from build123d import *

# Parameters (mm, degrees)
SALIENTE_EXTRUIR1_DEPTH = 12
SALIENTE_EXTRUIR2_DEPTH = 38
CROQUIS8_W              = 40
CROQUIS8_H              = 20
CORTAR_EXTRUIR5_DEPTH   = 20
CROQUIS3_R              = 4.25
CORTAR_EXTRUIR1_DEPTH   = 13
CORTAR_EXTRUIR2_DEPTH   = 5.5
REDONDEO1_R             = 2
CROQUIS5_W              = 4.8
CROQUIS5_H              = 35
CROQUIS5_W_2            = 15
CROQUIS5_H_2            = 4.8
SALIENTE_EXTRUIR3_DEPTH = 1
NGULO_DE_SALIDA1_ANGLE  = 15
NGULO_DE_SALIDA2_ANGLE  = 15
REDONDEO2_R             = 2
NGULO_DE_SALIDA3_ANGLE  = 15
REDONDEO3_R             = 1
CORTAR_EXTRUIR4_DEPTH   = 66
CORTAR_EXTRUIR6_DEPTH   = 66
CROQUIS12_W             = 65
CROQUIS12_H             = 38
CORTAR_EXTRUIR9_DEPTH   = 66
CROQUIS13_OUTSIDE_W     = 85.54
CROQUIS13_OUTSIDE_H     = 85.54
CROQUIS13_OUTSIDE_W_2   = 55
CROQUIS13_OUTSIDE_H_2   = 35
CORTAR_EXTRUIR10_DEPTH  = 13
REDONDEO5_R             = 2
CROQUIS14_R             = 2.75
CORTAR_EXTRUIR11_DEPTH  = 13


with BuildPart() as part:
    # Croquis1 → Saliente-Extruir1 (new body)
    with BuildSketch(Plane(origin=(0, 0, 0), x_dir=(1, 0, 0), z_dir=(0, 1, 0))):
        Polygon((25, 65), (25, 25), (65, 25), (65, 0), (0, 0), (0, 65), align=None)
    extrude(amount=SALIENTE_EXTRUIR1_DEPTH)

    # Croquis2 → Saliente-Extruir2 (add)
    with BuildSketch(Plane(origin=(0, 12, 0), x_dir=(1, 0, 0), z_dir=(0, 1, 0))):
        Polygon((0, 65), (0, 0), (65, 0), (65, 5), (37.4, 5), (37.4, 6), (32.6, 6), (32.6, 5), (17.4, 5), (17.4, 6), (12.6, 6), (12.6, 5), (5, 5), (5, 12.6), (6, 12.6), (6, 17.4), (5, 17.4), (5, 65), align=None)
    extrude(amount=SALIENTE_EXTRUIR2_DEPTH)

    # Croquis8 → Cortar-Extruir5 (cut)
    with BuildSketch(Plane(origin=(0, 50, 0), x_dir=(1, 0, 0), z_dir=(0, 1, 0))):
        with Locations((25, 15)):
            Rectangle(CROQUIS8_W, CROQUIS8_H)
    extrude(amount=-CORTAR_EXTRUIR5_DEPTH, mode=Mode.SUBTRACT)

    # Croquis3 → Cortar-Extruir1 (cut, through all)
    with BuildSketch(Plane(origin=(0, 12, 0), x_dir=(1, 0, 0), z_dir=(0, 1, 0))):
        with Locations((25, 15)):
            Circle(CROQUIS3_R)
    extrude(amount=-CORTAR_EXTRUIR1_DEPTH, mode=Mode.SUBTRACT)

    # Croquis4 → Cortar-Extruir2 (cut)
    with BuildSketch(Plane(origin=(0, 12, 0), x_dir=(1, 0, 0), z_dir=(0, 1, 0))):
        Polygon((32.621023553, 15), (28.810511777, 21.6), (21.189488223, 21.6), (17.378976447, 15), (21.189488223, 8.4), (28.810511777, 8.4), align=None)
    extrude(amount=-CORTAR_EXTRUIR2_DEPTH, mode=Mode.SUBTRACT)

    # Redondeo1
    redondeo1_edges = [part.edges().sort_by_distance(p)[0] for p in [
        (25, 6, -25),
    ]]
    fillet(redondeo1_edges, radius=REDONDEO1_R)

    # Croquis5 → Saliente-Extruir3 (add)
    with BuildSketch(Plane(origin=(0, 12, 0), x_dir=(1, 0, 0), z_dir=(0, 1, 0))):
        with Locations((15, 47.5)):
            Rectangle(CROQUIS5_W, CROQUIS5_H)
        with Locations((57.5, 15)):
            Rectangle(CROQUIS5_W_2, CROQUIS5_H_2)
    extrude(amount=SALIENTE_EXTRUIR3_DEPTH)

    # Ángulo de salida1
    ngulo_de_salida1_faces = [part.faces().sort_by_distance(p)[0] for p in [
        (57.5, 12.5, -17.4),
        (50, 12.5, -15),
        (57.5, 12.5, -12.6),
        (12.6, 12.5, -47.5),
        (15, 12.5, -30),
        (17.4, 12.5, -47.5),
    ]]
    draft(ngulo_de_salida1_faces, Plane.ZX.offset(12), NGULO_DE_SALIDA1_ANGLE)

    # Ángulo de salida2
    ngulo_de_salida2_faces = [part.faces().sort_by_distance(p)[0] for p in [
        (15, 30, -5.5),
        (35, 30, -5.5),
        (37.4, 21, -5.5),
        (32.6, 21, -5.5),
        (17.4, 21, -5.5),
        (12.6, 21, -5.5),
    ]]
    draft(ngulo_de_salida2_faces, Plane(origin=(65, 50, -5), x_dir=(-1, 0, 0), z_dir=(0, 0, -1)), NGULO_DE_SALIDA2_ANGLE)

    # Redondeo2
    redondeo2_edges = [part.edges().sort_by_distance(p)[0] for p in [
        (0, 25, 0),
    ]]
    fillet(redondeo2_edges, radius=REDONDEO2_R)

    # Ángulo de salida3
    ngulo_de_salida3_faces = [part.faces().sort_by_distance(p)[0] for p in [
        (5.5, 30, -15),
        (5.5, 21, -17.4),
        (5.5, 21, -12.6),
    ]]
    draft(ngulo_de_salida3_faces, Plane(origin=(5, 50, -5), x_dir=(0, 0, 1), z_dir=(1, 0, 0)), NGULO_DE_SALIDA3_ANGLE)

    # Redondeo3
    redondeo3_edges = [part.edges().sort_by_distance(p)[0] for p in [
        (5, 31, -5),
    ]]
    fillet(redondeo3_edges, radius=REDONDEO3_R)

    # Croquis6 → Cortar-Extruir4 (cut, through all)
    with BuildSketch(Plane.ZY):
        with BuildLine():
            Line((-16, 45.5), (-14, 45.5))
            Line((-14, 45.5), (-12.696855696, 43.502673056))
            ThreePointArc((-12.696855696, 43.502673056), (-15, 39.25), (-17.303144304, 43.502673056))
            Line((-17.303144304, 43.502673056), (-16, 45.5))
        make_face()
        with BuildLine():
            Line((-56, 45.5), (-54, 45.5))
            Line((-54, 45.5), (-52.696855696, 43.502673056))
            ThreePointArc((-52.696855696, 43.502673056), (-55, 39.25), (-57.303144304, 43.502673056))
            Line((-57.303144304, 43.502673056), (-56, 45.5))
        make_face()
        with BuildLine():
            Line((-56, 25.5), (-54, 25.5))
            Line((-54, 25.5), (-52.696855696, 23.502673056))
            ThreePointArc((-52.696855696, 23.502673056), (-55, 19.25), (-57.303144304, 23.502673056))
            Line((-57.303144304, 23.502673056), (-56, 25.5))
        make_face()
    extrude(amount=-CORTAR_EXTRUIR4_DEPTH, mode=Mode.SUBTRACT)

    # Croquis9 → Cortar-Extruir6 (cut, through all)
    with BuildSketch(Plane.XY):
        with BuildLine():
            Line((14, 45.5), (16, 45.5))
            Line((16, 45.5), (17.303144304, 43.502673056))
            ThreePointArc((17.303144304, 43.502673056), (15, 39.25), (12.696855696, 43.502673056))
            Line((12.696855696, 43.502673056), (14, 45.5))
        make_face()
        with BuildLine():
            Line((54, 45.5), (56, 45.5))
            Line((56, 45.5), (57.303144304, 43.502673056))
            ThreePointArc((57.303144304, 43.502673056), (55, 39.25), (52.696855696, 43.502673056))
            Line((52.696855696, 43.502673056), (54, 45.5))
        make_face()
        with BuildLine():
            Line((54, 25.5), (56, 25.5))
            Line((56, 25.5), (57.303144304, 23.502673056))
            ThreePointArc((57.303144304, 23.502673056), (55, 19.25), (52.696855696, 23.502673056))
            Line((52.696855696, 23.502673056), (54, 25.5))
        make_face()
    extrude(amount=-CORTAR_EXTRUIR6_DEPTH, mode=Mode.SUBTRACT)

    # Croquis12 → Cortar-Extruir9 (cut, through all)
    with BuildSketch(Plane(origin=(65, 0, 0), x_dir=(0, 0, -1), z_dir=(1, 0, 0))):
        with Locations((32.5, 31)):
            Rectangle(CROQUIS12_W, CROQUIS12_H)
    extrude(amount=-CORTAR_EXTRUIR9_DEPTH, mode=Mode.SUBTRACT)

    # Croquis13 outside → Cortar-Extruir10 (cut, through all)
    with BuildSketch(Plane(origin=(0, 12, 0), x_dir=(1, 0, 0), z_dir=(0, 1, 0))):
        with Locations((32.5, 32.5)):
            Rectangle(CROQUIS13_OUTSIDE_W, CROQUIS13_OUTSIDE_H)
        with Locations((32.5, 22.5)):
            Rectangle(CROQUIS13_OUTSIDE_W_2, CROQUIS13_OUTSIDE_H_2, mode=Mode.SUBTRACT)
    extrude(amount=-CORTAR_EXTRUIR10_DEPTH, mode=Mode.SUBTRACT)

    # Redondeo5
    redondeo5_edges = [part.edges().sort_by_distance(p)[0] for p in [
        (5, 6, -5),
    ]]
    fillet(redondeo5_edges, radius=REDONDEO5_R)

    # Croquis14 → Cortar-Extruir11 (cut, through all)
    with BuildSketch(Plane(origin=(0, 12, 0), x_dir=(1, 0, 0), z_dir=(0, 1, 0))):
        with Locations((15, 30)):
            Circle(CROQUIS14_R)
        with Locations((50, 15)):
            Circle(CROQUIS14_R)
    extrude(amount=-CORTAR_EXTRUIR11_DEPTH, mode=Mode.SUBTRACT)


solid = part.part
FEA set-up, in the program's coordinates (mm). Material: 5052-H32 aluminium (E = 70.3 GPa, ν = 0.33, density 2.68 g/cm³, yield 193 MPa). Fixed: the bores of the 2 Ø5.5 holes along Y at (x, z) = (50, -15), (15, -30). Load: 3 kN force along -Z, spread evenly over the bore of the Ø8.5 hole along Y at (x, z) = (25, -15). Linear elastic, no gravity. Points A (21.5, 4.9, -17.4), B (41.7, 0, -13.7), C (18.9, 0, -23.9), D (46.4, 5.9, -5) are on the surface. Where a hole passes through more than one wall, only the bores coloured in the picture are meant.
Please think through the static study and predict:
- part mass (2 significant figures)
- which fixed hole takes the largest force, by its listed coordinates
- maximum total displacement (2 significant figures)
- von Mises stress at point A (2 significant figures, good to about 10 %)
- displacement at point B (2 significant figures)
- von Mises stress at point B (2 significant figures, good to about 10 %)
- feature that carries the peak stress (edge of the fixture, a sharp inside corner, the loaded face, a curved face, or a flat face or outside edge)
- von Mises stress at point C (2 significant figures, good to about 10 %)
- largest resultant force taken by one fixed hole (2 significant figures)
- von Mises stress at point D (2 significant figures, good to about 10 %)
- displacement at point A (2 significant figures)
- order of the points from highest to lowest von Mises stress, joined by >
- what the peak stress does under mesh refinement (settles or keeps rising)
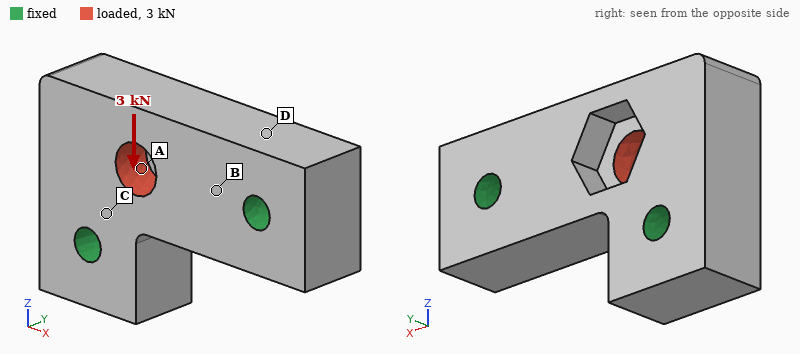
40 g
(15, -30)
11 µm
32 MPa
3.2 µm
14 MPa
edge of the fixture
24 MPa
2.3 kN
5.8 MPa
4.6 µm
A > C > B > D
keeps rising
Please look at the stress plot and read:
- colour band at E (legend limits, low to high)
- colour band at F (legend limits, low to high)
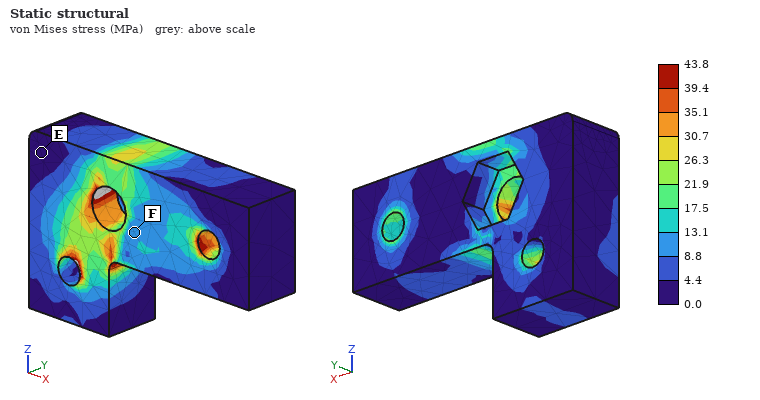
0.0 to 4.4 MPa
8.8 to 13.1 MPa
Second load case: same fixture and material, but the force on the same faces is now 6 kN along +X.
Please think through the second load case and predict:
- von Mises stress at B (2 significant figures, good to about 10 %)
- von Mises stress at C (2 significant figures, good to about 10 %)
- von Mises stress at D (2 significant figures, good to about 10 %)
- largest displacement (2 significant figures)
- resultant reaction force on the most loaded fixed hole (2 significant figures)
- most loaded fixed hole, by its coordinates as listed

34 MPa
24 MPa
9.0 MPa
15 µm
4.1 kN
(50, -15)
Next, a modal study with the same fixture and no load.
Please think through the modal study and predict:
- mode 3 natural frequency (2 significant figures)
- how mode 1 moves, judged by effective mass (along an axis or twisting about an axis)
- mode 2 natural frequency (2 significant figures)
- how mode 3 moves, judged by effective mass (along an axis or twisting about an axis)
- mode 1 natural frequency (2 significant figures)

28 kHz
along Y
27 kHz
along X
15 kHz
